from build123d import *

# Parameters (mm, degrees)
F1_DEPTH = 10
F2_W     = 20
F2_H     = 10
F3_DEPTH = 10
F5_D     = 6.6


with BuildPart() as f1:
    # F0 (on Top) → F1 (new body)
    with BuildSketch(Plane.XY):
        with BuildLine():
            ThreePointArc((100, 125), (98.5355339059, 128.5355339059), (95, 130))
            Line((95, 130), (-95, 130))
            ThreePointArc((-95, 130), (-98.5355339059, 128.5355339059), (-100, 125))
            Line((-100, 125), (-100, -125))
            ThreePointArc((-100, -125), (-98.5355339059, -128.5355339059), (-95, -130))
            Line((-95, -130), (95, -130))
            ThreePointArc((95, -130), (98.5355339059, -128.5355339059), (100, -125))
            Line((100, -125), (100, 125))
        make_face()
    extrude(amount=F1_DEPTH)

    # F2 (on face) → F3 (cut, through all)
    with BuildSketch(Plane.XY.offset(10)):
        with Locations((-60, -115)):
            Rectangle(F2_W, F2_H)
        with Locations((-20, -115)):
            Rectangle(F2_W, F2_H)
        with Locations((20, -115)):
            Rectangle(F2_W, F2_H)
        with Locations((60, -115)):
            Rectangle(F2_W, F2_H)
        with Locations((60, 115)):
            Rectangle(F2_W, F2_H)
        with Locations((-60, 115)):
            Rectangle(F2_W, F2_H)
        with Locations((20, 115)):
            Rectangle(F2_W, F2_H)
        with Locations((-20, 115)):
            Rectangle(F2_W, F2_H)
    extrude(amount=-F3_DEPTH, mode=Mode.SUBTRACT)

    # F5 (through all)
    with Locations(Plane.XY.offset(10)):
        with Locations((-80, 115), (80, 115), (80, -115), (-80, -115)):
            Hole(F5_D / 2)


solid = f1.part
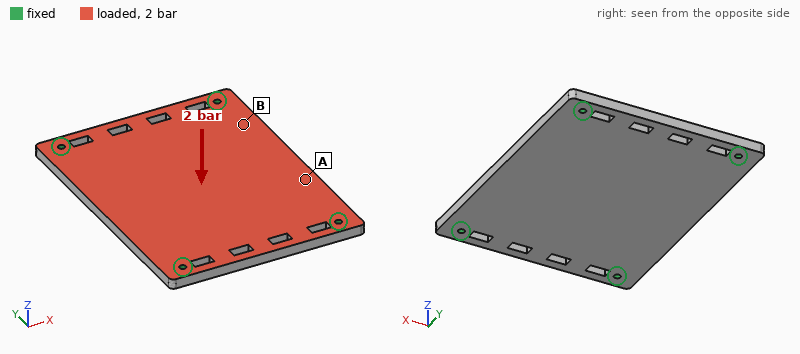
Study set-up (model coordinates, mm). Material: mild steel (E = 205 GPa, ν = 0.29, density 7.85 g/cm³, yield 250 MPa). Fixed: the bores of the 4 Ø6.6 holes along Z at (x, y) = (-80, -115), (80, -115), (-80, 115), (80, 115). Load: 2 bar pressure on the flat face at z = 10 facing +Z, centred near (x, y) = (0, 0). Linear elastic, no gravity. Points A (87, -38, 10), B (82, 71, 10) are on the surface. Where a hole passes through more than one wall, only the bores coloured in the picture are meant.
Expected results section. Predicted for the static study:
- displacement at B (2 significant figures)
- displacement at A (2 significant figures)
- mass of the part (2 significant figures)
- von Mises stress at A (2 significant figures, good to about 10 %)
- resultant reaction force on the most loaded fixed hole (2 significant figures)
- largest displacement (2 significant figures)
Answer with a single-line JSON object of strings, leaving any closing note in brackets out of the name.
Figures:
{"displacement at B": "0.066 mm", "displacement at A": "0.12 mm", "mass of the part": "3.9 kg", "von Mises stress at A": "30 MPa", "resultant reaction force on the most loaded fixed hole": "2.5 kN", "largest displacement": "0.17 mm"}
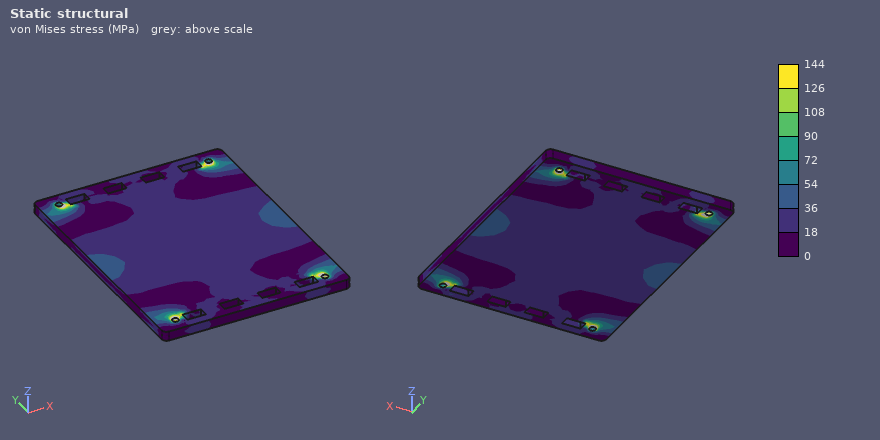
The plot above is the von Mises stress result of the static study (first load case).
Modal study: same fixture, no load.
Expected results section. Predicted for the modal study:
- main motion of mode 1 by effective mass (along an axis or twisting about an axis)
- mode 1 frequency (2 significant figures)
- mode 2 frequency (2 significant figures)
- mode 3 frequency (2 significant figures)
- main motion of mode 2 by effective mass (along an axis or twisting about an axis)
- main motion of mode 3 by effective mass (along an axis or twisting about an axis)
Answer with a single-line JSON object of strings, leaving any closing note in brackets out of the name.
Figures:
{"main motion of mode 1 by effective mass": "along Z", "mode 1 frequency": "720 Hz", "mode 2 frequency": "1100 Hz", "mode 3 frequency": "1700 Hz", "main motion of mode 2 by effective mass": "twisting about Y", "main motion of mode 3 by effective mass": "twisting about X"}
